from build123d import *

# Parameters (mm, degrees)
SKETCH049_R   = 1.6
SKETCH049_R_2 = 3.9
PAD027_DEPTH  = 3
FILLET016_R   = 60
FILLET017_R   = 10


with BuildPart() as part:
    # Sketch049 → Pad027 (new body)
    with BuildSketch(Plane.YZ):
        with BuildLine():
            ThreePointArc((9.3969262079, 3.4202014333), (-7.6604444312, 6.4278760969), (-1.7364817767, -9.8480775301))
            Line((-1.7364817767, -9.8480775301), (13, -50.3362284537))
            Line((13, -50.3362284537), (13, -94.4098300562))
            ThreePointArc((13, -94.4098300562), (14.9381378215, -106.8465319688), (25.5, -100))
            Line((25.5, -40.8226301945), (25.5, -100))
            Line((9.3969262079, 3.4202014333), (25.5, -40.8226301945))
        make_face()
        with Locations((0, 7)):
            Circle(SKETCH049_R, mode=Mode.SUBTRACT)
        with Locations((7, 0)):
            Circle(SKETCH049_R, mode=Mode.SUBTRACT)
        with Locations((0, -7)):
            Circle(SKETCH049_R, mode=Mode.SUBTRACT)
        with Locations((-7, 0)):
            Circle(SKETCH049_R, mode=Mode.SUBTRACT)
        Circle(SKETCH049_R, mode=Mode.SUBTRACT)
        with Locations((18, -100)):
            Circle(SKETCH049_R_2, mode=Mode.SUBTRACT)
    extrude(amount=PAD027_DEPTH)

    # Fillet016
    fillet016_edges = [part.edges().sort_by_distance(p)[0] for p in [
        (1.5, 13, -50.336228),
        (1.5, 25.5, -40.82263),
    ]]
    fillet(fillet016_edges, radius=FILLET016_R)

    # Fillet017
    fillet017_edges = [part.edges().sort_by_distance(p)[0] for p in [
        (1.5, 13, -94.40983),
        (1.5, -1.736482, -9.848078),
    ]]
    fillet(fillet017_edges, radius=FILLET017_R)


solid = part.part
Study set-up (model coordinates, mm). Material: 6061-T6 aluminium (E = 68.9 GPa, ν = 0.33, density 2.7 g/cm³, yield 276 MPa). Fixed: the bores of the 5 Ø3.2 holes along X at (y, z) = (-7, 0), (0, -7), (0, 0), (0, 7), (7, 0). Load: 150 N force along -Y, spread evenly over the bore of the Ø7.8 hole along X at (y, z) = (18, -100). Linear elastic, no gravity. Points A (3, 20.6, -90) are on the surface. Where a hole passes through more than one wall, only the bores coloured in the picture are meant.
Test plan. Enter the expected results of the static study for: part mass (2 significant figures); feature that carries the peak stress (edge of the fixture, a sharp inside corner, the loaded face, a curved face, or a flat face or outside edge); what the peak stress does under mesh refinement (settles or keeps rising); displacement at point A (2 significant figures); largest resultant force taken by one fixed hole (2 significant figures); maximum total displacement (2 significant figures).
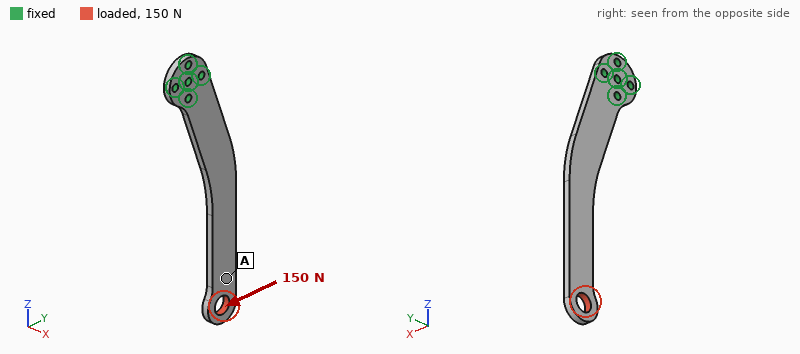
13 g
edge of the fixture
keeps rising
0.74 mm
1.2 kN
1.00 mm
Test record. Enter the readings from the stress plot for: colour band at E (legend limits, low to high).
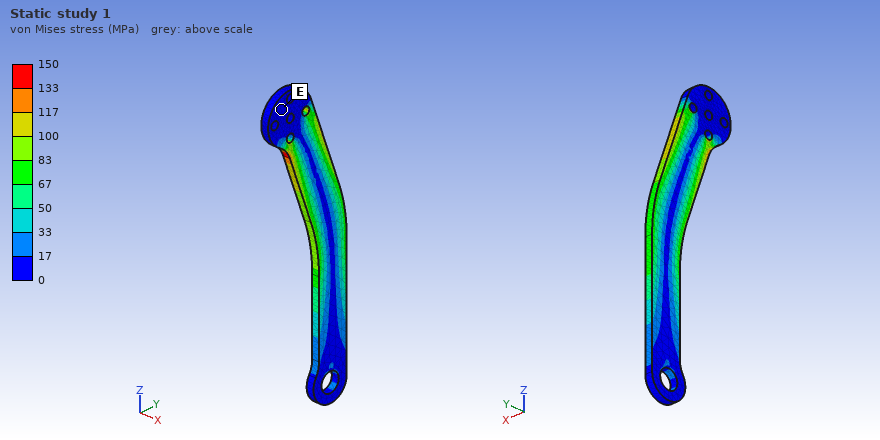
0 to 17 MPa
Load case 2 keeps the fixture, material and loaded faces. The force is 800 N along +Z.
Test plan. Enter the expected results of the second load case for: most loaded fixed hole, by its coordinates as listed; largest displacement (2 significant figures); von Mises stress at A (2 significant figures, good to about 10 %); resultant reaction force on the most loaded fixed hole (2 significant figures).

(7, 0)
0.32 mm
16 MPa
1.2 kN
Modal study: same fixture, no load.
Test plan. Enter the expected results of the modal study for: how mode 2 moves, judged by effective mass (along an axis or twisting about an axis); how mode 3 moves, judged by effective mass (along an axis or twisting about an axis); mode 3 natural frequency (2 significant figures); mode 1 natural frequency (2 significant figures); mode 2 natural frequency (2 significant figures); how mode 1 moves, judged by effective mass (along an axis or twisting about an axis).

along Y
along X
1400 Hz
260 Hz
1200 Hz
along X
